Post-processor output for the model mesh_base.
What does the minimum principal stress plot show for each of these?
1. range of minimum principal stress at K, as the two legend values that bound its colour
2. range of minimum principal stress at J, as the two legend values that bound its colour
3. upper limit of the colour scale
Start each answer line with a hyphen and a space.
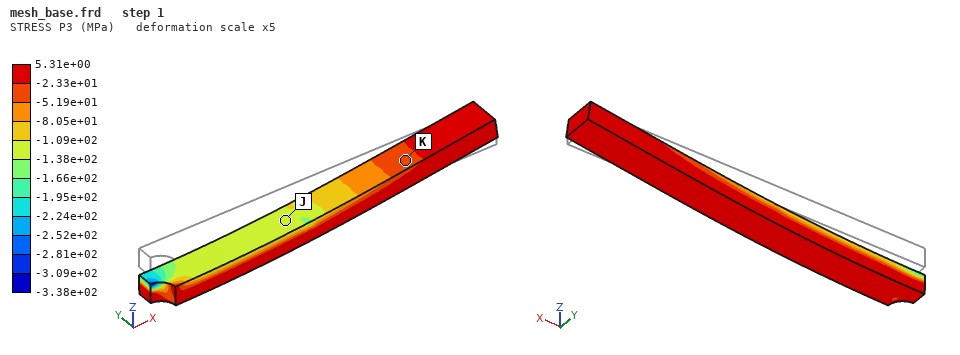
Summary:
- -5.19e+01 to -2.33e+01 MPa
- -1.38e+02 to -1.09e+02 MPa
- 5.31e+00 MPa
